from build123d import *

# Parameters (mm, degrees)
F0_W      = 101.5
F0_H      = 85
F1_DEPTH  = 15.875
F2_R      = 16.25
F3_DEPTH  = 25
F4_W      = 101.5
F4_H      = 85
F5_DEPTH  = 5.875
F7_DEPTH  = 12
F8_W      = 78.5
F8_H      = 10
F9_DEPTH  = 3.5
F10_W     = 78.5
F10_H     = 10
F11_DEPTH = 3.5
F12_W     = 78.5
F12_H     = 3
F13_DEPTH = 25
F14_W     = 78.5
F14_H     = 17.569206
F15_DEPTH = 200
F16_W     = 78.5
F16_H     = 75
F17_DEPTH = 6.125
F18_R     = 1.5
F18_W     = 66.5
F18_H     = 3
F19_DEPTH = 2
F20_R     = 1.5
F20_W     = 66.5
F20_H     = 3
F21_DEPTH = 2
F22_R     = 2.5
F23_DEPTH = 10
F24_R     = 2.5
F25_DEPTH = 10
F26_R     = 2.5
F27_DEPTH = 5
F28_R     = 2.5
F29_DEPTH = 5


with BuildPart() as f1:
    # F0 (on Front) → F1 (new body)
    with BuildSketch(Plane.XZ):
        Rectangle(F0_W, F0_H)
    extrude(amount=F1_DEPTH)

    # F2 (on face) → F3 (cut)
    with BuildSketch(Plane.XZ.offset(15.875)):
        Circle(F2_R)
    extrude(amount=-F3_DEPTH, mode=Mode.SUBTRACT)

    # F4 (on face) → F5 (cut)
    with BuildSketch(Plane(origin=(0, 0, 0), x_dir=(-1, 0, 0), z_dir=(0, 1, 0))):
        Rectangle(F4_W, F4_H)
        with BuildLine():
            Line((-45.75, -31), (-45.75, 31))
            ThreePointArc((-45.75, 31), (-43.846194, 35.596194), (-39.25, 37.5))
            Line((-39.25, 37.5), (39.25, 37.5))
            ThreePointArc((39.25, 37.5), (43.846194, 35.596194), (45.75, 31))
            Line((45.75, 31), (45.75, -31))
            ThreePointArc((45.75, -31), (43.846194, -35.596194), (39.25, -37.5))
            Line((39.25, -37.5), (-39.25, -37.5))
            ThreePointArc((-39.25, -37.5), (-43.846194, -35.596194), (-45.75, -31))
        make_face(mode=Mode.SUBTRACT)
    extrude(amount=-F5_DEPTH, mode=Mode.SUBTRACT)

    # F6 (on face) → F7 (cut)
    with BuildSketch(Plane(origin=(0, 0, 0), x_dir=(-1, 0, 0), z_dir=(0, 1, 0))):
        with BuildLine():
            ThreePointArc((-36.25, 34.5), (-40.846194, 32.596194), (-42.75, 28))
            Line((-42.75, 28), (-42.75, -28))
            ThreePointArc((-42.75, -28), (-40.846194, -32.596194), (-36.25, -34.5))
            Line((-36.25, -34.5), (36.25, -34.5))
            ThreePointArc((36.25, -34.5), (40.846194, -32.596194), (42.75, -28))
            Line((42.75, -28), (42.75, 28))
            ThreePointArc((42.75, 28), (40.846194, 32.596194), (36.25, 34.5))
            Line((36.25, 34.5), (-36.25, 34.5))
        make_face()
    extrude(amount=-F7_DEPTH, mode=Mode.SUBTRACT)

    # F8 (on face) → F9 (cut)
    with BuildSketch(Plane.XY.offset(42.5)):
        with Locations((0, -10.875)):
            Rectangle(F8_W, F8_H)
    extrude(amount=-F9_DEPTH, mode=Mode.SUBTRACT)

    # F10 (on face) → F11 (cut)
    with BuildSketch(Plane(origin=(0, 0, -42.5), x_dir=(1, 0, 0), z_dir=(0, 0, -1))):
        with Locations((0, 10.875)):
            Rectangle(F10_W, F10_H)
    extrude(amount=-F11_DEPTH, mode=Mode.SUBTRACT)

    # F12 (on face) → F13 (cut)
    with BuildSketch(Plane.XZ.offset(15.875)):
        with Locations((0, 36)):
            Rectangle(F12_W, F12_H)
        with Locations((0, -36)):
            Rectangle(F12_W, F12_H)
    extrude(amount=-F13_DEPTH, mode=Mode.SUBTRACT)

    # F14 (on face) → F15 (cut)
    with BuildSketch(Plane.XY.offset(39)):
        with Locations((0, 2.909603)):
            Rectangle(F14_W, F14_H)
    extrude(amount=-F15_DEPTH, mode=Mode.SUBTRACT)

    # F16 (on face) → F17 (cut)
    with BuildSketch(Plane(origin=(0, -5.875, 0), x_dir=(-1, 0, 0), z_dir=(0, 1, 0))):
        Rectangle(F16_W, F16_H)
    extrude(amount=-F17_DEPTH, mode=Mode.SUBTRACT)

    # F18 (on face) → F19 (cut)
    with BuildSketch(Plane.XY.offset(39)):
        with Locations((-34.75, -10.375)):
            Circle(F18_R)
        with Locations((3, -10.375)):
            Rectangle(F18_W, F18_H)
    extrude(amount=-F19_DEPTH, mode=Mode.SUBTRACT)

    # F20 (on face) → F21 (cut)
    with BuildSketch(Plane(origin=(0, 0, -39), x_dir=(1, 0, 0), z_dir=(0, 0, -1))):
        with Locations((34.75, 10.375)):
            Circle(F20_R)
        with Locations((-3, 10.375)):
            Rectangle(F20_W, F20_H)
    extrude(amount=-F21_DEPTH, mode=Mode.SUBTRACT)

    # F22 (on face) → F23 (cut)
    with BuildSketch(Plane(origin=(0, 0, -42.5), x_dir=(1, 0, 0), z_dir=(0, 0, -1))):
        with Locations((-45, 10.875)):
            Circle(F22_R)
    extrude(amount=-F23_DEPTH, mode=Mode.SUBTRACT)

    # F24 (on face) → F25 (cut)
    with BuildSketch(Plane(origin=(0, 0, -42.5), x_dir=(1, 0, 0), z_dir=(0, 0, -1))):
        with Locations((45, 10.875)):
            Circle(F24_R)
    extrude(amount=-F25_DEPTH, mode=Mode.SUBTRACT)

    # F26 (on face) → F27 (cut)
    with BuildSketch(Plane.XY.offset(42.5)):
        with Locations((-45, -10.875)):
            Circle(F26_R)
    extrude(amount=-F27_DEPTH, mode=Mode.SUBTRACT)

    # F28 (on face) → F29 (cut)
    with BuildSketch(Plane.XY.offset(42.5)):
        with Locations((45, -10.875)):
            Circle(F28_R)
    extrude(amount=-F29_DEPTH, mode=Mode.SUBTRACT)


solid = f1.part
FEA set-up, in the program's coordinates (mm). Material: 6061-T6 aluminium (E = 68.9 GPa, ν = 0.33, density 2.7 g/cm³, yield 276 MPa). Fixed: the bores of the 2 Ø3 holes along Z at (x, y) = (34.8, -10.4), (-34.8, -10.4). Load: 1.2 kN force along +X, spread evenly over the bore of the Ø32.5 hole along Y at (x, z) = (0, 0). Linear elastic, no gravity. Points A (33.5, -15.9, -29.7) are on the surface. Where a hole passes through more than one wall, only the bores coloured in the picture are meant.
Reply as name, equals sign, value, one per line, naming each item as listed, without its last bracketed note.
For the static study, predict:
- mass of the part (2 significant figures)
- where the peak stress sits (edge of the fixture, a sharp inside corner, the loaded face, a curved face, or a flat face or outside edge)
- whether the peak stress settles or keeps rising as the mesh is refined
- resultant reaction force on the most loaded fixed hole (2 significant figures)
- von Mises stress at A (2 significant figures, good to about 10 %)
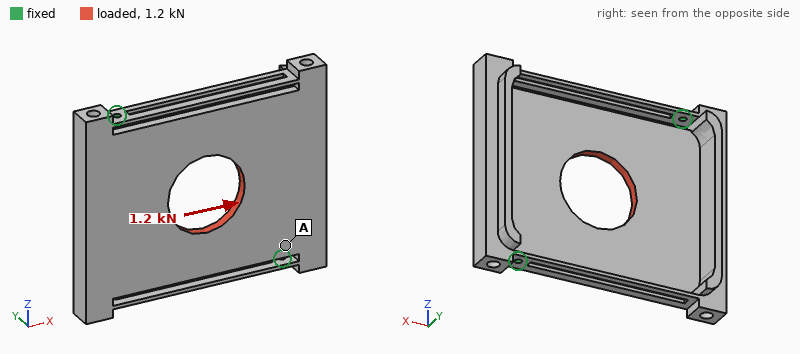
mass of the part = 100 g
where the peak stress sits = edge of the fixture
whether the peak stress settles or keeps rising as the mesh is refined = keeps rising
resultant reaction force on the most loaded fixed hole = 600 N
von Mises stress at A = 11 MPa
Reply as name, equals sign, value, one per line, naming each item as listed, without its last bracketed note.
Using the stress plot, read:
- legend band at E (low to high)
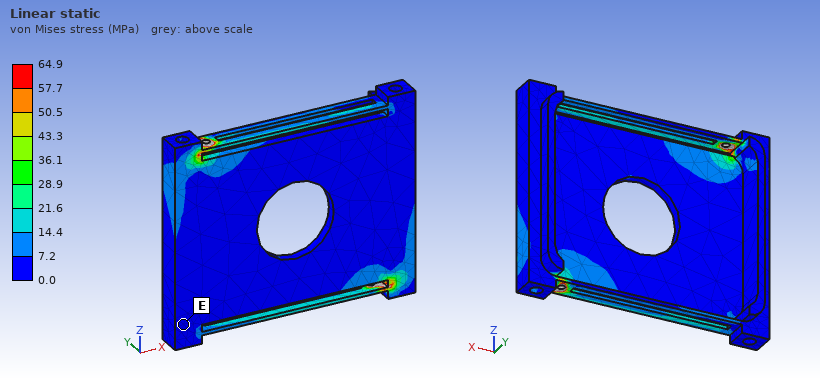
legend band at E = 0.0 to 7.2 MPa
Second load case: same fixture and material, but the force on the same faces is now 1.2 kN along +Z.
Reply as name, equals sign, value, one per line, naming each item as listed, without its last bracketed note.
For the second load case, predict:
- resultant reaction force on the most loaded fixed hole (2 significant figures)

resultant reaction force on the most loaded fixed hole = 600 N
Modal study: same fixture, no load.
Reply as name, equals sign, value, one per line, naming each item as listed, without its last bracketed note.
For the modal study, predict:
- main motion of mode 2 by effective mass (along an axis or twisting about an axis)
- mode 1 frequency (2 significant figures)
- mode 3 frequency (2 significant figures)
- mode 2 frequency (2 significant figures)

main motion of mode 2 by effective mass = along Y
mode 1 frequency = 380 Hz
mode 3 frequency = 1500 Hz
mode 2 frequency = 580 Hz
